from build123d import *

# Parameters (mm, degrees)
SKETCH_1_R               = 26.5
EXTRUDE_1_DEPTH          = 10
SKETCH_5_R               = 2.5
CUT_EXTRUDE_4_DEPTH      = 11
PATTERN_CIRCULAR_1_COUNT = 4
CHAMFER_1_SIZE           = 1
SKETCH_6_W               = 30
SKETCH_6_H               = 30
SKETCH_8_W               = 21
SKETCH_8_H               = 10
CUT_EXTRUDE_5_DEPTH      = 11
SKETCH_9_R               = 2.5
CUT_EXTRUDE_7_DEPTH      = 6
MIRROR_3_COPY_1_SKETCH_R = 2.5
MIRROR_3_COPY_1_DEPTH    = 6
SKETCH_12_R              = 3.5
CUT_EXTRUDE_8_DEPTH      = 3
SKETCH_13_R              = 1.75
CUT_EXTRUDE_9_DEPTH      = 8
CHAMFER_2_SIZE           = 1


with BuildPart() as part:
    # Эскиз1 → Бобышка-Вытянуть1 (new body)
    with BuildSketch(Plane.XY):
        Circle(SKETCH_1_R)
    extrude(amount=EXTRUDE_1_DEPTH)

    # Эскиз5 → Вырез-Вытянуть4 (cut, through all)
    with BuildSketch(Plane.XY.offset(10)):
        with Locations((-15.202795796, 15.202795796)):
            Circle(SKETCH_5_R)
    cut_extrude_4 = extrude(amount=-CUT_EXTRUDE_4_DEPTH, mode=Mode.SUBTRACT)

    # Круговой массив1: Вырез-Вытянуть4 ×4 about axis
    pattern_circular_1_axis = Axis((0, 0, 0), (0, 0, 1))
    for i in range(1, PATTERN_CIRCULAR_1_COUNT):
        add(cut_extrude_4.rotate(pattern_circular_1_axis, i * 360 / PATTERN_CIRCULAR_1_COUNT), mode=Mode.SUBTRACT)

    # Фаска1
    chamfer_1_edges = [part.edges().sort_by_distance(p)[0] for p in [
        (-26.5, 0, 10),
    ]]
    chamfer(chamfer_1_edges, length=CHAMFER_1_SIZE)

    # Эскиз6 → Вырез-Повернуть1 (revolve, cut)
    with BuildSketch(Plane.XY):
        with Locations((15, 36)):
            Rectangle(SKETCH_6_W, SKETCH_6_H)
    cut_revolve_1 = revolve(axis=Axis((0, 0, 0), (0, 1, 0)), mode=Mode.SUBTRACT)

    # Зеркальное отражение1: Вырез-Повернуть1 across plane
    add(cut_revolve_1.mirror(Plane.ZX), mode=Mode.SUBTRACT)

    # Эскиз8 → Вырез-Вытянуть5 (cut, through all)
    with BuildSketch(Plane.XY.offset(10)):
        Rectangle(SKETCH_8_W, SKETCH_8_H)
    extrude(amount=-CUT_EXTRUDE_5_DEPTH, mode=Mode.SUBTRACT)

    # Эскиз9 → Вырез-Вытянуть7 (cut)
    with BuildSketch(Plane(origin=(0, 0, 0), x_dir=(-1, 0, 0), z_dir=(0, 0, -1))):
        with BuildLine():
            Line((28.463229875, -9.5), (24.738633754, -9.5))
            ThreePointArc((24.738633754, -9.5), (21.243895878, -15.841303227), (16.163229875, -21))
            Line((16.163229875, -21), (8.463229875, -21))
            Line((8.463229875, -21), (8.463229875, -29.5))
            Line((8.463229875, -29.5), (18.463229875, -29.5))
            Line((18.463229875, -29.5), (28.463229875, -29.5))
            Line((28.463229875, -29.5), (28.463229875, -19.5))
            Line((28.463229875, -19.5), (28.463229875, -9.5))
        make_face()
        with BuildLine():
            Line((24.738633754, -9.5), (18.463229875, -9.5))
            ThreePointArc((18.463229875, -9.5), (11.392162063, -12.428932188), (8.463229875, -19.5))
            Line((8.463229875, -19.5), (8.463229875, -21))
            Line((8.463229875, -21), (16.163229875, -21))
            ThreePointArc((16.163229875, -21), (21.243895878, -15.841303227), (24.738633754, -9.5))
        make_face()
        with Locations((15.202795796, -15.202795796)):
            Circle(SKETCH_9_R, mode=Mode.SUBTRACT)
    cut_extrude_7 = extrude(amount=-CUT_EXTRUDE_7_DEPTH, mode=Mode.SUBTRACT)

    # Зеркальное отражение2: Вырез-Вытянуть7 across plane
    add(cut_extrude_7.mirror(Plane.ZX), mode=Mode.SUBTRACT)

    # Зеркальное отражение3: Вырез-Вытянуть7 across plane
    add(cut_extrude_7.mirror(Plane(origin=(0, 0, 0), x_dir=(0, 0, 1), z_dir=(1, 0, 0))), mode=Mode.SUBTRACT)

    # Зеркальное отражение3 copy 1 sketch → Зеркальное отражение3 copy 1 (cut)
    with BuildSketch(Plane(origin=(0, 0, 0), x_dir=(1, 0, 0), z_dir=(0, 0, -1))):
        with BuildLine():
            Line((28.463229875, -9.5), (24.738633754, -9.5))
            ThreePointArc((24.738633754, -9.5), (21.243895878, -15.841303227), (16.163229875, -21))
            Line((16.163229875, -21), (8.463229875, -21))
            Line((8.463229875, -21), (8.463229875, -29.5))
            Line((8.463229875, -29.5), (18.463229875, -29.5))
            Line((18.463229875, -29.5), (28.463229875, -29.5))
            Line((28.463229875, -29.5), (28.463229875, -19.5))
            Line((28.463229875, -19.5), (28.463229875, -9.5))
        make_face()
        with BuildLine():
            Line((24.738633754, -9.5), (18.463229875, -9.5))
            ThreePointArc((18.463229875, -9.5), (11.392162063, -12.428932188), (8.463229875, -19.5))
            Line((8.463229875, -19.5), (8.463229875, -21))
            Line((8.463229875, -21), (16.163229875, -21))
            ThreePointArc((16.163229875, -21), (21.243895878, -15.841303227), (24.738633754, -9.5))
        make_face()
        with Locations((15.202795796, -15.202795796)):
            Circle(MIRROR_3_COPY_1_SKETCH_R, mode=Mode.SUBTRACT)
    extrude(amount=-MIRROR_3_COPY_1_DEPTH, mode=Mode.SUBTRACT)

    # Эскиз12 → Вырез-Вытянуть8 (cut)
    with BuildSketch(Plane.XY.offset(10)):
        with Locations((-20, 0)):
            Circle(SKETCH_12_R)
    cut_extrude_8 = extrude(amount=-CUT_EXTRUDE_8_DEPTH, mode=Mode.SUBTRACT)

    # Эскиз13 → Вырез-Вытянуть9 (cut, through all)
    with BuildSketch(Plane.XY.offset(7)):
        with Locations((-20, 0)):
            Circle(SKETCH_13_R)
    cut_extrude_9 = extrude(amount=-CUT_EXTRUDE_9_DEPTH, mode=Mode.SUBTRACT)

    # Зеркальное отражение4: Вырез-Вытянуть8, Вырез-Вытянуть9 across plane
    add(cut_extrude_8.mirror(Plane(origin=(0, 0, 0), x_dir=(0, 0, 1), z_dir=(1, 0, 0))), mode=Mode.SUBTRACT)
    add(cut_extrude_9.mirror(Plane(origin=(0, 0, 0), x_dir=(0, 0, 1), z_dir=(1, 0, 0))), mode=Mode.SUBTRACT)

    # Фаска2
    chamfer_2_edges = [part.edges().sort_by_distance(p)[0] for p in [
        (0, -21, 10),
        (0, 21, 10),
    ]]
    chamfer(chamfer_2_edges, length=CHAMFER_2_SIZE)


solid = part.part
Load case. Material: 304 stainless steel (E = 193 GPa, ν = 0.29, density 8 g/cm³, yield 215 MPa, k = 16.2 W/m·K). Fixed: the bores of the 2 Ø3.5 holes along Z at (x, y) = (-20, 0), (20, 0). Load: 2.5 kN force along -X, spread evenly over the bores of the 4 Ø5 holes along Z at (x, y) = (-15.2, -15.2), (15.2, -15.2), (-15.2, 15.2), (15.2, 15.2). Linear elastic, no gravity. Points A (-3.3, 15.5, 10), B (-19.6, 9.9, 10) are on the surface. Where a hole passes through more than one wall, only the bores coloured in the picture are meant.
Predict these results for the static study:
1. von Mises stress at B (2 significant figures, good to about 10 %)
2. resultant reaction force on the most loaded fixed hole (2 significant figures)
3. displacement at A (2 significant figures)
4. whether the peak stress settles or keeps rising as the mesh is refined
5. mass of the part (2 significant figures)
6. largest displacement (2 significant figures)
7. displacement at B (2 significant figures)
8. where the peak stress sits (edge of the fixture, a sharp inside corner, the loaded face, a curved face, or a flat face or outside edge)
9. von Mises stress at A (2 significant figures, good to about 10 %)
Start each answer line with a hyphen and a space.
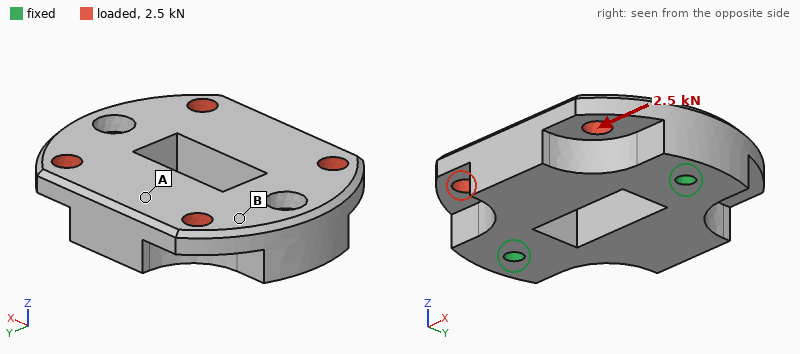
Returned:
- 5.2 MPa
- 1.3 kN
- 1.2 µm
- keeps rising
- 110 g
- 2.1 µm
- 1.0 µm
- edge of the fixture
- 8.6 MPa
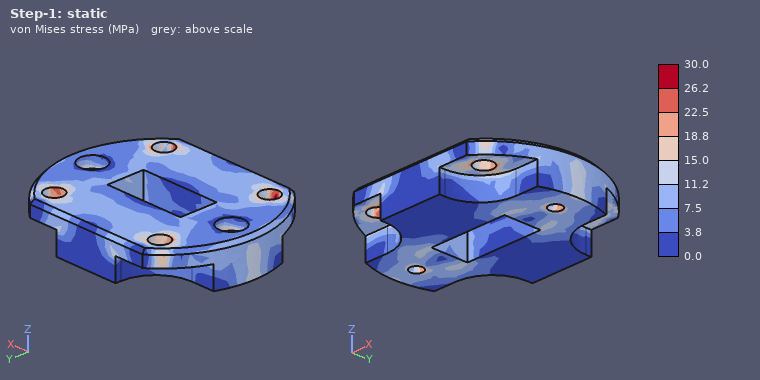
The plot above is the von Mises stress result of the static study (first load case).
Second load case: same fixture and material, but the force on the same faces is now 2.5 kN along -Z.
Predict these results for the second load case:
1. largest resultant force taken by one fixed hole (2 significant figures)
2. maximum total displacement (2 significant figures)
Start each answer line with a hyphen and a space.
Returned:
- 1.3 kN
- 13 µm
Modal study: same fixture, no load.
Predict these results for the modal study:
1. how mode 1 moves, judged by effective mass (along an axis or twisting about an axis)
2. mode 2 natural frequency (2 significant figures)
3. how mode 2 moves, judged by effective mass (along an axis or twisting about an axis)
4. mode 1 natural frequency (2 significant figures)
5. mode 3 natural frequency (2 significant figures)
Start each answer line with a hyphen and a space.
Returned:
- twisting about X
- 11 kHz
- along Z
- 8000 Hz
- 21 kHz
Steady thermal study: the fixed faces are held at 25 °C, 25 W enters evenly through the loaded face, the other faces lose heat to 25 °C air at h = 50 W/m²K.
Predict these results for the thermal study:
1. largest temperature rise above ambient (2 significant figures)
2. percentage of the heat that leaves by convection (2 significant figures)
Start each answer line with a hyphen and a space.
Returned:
- 72 K
- 34 %
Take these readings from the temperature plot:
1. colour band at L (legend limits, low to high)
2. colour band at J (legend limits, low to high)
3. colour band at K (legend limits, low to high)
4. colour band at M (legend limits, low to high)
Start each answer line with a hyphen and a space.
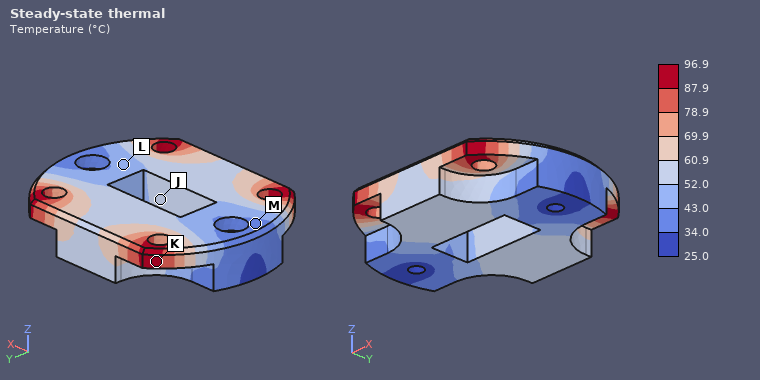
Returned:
- 43.0 to 52.0 °C
- 52.0 to 60.9 °C
- 87.9 to 96.9 °C
- 34.0 to 43.0 °C
